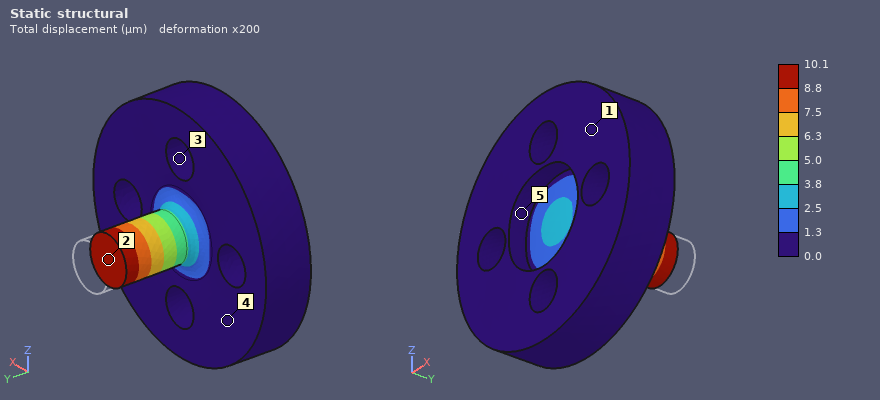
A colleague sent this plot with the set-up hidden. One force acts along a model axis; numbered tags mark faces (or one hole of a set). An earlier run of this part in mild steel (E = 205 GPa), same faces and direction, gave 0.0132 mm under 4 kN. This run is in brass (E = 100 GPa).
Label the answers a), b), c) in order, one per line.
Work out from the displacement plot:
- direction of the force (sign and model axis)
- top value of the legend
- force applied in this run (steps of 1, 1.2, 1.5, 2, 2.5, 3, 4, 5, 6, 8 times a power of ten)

a) -Y
b) 10.1 µm
c) 1.5 kN
